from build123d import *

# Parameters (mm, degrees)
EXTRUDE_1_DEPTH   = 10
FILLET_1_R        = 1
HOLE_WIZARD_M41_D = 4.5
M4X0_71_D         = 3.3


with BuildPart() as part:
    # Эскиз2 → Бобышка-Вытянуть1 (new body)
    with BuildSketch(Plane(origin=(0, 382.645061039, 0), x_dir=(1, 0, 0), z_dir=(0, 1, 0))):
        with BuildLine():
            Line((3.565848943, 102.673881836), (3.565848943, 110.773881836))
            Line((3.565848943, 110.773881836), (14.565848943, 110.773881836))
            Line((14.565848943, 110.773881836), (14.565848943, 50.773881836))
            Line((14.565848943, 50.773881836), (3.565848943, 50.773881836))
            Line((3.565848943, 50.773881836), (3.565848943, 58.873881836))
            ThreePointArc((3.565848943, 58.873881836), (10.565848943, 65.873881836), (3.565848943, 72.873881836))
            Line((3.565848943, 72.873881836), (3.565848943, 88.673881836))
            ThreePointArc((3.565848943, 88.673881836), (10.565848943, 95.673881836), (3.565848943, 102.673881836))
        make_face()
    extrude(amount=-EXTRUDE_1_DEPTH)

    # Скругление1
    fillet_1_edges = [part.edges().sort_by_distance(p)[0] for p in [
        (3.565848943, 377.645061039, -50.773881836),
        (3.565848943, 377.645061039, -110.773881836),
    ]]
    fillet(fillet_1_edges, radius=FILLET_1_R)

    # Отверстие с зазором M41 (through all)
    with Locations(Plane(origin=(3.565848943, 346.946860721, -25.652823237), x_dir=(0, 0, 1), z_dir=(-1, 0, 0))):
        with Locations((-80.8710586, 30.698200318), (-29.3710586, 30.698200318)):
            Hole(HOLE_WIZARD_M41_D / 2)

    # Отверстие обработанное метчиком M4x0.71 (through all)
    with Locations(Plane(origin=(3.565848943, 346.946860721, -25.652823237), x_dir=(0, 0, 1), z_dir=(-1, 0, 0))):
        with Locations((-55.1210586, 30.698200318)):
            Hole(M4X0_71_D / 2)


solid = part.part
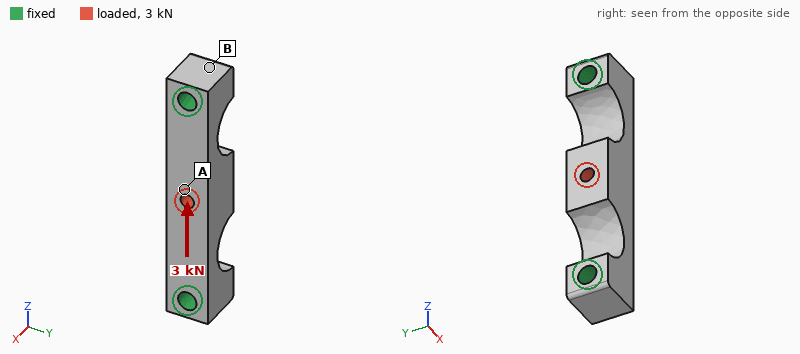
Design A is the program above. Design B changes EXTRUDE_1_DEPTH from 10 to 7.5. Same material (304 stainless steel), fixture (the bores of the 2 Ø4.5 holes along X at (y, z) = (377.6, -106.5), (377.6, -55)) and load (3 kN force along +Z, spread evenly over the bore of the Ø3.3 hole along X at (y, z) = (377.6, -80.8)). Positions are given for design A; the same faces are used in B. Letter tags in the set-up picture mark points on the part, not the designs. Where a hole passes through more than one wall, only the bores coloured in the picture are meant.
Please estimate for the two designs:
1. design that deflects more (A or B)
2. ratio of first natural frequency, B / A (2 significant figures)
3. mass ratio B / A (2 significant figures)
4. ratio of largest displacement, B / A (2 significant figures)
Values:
B
0.91
0.73
1.5
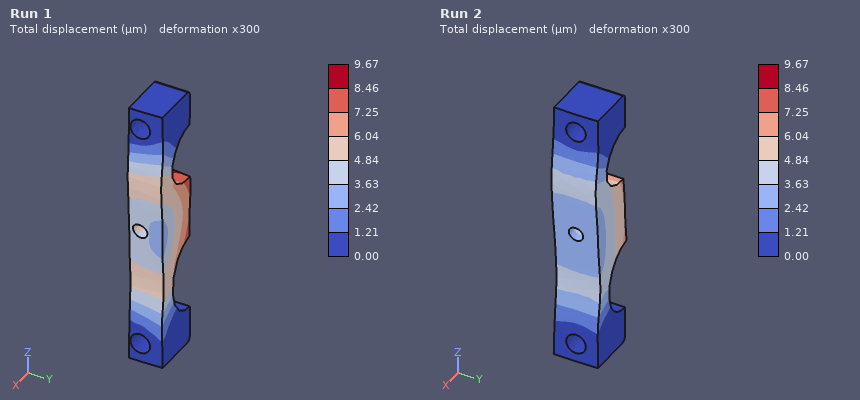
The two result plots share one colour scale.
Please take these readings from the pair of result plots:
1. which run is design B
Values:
Run 1
